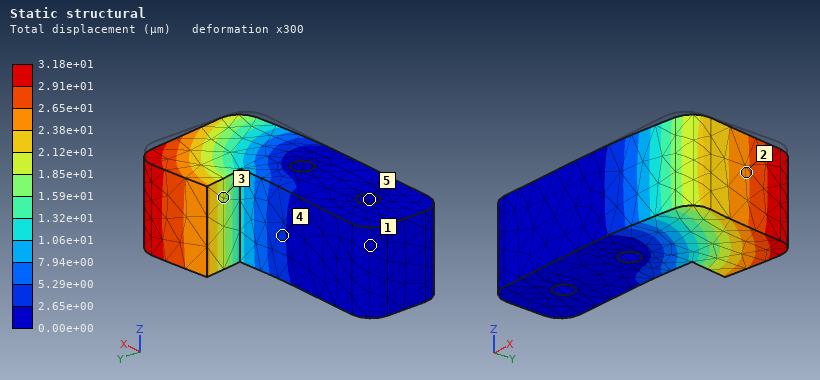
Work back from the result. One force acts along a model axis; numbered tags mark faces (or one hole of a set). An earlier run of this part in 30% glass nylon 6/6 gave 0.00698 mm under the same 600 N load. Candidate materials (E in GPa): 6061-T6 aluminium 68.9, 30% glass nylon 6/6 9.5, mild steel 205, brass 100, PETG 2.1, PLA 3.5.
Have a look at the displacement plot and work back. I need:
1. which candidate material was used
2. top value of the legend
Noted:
PETG
3.18e+01 µm
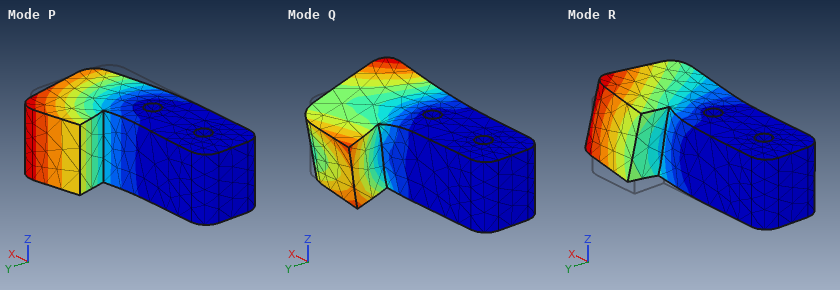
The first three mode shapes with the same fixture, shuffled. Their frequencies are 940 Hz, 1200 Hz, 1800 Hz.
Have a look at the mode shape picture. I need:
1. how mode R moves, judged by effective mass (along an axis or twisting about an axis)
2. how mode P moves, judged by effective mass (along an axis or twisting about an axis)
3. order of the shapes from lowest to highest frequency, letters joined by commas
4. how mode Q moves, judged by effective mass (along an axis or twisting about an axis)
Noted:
along Z
along Y
P, R, Q
twisting about X
